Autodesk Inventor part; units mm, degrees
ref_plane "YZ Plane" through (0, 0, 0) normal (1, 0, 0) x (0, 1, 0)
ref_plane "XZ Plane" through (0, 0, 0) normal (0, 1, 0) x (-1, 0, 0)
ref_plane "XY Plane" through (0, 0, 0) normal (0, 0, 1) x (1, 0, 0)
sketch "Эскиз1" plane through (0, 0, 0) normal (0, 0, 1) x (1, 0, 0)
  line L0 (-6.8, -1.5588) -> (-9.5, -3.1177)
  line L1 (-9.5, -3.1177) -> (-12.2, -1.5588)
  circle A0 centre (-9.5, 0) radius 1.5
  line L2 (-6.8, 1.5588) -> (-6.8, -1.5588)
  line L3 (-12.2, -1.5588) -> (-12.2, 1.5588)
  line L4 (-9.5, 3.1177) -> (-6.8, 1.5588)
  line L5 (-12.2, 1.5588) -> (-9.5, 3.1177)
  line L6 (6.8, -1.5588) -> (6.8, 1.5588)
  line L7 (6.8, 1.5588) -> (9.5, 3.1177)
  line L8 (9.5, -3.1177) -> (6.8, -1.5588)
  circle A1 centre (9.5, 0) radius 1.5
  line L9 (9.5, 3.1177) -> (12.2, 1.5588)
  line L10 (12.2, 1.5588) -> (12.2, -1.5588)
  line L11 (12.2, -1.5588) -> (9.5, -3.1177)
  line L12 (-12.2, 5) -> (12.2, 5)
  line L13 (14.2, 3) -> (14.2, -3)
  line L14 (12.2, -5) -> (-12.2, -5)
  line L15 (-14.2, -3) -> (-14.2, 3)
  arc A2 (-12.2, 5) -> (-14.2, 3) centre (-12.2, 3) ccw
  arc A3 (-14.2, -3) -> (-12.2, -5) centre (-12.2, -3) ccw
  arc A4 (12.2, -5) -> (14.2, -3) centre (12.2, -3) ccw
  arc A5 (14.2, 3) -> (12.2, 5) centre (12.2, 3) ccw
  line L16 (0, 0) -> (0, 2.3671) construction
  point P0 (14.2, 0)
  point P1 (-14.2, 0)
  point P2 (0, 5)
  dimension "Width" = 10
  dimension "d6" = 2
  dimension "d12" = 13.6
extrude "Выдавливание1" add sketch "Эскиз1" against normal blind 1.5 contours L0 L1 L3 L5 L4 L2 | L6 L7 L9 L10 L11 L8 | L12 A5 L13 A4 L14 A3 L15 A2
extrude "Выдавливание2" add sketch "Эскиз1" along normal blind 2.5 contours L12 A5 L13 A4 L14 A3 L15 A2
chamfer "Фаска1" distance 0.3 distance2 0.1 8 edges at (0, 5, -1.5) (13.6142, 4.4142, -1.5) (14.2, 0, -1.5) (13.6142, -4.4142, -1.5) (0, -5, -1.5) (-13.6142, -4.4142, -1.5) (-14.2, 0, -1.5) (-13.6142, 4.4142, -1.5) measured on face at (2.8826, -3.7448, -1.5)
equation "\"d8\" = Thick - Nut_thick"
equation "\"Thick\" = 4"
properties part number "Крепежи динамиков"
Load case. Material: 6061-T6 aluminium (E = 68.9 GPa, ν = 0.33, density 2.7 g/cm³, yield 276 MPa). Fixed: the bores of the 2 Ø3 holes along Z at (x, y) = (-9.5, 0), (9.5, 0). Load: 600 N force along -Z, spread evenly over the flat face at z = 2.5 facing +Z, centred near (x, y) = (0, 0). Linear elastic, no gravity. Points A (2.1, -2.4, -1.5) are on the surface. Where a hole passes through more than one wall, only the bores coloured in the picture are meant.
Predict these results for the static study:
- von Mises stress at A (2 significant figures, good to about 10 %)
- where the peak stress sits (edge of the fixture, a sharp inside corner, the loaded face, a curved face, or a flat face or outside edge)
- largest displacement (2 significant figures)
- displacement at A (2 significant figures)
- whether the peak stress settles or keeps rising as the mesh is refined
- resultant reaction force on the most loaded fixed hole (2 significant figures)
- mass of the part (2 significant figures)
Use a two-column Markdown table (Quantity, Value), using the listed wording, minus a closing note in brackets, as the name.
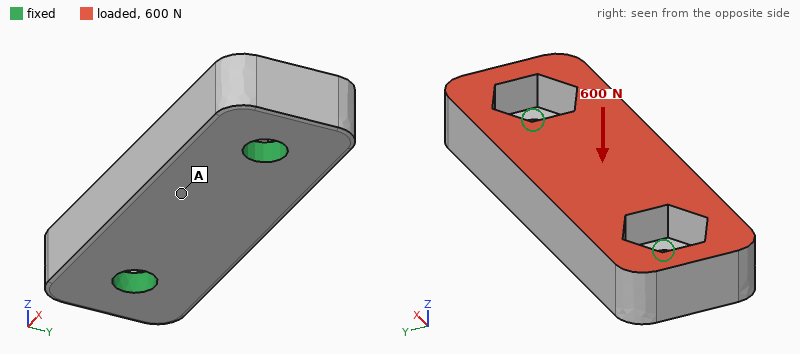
| Quantity | Value |
|---|---|
| von Mises stress at A | 13 MPa |
| where the peak stress sits | edge of the fixture |
| largest displacement | 6.4 µm |
| displacement at A | 5.6 µm |
| whether the peak stress settles or keeps rising as the mesh is refined | keeps rising |
| resultant reaction force on the most loaded fixed hole | 330 N |
| mass of the part | 2.6 g |
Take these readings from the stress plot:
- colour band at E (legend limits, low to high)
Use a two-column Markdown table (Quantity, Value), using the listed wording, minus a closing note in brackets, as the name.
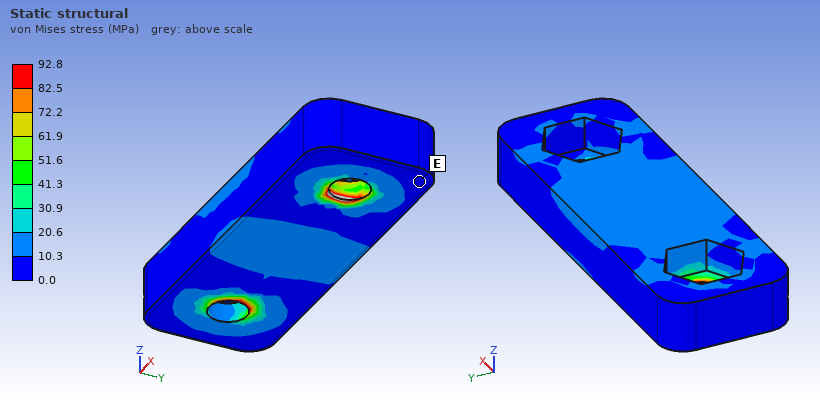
| Quantity | Value |
|---|---|
| colour band at E | 0.0 to 10.3 MPa |
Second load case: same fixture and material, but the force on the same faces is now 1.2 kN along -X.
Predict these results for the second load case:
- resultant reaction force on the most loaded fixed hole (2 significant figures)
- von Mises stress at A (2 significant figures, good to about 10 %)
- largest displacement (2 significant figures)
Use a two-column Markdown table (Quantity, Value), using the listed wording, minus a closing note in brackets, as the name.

| Quantity | Value |
|---|---|
| resultant reaction force on the most loaded fixed hole | 630 N |
| von Mises stress at A | 11 MPa |
| largest displacement | 8.2 µm |
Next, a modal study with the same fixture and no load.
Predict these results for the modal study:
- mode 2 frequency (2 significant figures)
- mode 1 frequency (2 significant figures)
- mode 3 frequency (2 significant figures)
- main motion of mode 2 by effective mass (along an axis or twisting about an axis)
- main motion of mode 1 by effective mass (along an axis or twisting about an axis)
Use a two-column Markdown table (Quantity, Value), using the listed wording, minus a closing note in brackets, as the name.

| Quantity | Value |
|---|---|
| mode 2 frequency | 34 kHz |
| mode 1 frequency | 27 kHz |
| mode 3 frequency | 48 kHz |
| main motion of mode 2 by effective mass | along Z |
| main motion of mode 1 by effective mass | along Y |
